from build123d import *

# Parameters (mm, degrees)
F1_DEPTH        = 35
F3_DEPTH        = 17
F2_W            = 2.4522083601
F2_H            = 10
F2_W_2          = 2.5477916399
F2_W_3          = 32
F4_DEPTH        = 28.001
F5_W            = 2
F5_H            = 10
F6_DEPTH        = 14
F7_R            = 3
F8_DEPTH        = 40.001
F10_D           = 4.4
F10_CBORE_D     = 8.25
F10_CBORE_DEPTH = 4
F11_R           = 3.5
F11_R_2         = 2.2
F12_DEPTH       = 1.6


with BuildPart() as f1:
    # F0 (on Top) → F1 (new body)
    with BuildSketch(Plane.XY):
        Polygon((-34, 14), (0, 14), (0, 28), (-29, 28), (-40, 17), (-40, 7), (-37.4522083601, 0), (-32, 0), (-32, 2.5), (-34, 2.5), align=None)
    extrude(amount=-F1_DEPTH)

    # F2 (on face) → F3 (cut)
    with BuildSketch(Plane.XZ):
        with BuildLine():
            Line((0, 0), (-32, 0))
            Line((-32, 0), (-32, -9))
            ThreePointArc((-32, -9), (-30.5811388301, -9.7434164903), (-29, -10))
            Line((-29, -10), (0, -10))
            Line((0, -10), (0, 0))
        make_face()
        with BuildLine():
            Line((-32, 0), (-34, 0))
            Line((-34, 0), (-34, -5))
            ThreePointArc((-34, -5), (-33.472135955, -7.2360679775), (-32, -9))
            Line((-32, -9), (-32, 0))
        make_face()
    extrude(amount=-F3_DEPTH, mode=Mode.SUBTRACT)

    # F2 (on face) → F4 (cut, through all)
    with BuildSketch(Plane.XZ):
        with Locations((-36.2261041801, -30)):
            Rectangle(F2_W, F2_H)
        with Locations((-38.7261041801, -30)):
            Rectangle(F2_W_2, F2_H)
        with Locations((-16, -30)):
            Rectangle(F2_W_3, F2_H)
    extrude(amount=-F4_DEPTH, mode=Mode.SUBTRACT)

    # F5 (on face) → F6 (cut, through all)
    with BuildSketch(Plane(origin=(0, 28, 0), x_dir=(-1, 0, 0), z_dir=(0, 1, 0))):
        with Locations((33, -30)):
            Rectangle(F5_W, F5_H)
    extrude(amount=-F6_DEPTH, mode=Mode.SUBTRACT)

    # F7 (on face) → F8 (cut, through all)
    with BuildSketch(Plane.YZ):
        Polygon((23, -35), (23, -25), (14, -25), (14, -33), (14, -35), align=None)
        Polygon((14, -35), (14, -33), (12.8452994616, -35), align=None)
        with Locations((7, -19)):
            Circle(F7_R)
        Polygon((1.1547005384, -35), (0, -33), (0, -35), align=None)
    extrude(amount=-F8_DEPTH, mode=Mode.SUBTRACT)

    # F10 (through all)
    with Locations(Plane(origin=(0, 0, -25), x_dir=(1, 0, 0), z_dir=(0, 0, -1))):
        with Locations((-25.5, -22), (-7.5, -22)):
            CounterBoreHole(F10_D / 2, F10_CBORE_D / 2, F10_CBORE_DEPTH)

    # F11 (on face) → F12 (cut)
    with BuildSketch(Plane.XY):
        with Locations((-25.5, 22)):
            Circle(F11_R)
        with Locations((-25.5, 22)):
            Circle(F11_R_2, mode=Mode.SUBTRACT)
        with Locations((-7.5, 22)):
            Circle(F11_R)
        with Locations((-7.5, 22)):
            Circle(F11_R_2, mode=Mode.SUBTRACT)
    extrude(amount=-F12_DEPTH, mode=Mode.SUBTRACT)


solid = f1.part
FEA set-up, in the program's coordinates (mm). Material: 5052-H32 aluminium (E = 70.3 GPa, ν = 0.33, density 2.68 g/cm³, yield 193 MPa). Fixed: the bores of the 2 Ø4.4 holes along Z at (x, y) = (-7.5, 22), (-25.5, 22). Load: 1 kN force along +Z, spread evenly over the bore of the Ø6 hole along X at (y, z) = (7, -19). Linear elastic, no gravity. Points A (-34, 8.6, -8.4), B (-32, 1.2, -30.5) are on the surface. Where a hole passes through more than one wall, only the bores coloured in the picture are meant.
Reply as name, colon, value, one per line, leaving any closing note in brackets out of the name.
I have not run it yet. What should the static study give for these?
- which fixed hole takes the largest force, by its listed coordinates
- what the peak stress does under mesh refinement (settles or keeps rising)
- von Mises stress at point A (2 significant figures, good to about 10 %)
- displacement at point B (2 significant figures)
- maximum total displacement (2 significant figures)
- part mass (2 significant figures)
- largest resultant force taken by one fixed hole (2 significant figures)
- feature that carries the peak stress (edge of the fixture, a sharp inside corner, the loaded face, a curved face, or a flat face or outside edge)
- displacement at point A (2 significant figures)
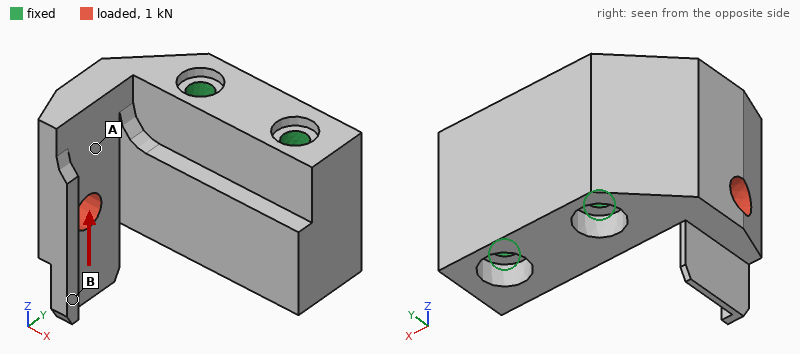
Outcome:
which fixed hole takes the largest force, by its listed coordinates: (-25.5, 22)
what the peak stress does under mesh refinement: keeps rising
von Mises stress at point A: 14 MPa
displacement at point B: 24 µm
maximum total displacement: 28 µm
part mass: 33 g
largest resultant force taken by one fixed hole: 1.1 kN
feature that carries the peak stress: edge of the fixture
displacement at point A: 13 µm
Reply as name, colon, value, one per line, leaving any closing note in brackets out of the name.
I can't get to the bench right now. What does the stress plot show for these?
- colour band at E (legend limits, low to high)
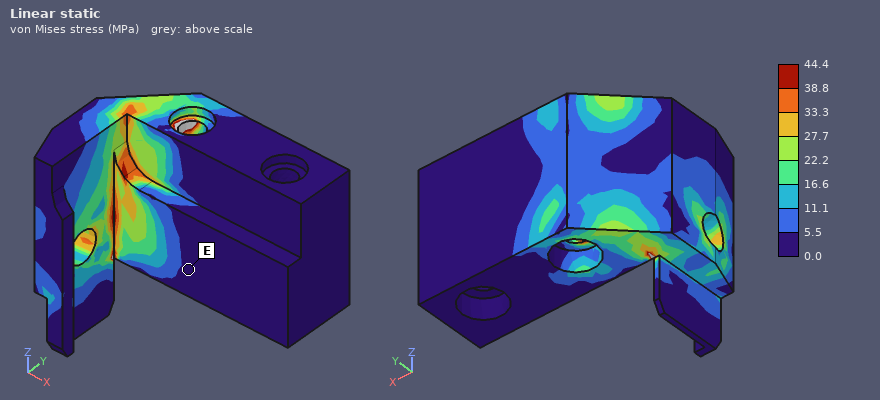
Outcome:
colour band at E: 0.0 to 5.5 MPa
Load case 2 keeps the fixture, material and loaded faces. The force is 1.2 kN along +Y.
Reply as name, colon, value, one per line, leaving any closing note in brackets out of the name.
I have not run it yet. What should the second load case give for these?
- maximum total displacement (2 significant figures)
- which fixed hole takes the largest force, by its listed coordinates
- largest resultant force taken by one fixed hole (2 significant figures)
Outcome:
maximum total displacement: 29 µm
which fixed hole takes the largest force, by its listed coordinates: (-25.5, 22)
largest resultant force taken by one fixed hole: 1.6 kN
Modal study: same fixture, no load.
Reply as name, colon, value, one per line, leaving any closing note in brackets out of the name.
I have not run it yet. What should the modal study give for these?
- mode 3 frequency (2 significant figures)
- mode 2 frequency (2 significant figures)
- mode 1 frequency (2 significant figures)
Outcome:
mode 3 frequency: 14 kHz
mode 2 frequency: 11 kHz
mode 1 frequency: 9900 Hz
